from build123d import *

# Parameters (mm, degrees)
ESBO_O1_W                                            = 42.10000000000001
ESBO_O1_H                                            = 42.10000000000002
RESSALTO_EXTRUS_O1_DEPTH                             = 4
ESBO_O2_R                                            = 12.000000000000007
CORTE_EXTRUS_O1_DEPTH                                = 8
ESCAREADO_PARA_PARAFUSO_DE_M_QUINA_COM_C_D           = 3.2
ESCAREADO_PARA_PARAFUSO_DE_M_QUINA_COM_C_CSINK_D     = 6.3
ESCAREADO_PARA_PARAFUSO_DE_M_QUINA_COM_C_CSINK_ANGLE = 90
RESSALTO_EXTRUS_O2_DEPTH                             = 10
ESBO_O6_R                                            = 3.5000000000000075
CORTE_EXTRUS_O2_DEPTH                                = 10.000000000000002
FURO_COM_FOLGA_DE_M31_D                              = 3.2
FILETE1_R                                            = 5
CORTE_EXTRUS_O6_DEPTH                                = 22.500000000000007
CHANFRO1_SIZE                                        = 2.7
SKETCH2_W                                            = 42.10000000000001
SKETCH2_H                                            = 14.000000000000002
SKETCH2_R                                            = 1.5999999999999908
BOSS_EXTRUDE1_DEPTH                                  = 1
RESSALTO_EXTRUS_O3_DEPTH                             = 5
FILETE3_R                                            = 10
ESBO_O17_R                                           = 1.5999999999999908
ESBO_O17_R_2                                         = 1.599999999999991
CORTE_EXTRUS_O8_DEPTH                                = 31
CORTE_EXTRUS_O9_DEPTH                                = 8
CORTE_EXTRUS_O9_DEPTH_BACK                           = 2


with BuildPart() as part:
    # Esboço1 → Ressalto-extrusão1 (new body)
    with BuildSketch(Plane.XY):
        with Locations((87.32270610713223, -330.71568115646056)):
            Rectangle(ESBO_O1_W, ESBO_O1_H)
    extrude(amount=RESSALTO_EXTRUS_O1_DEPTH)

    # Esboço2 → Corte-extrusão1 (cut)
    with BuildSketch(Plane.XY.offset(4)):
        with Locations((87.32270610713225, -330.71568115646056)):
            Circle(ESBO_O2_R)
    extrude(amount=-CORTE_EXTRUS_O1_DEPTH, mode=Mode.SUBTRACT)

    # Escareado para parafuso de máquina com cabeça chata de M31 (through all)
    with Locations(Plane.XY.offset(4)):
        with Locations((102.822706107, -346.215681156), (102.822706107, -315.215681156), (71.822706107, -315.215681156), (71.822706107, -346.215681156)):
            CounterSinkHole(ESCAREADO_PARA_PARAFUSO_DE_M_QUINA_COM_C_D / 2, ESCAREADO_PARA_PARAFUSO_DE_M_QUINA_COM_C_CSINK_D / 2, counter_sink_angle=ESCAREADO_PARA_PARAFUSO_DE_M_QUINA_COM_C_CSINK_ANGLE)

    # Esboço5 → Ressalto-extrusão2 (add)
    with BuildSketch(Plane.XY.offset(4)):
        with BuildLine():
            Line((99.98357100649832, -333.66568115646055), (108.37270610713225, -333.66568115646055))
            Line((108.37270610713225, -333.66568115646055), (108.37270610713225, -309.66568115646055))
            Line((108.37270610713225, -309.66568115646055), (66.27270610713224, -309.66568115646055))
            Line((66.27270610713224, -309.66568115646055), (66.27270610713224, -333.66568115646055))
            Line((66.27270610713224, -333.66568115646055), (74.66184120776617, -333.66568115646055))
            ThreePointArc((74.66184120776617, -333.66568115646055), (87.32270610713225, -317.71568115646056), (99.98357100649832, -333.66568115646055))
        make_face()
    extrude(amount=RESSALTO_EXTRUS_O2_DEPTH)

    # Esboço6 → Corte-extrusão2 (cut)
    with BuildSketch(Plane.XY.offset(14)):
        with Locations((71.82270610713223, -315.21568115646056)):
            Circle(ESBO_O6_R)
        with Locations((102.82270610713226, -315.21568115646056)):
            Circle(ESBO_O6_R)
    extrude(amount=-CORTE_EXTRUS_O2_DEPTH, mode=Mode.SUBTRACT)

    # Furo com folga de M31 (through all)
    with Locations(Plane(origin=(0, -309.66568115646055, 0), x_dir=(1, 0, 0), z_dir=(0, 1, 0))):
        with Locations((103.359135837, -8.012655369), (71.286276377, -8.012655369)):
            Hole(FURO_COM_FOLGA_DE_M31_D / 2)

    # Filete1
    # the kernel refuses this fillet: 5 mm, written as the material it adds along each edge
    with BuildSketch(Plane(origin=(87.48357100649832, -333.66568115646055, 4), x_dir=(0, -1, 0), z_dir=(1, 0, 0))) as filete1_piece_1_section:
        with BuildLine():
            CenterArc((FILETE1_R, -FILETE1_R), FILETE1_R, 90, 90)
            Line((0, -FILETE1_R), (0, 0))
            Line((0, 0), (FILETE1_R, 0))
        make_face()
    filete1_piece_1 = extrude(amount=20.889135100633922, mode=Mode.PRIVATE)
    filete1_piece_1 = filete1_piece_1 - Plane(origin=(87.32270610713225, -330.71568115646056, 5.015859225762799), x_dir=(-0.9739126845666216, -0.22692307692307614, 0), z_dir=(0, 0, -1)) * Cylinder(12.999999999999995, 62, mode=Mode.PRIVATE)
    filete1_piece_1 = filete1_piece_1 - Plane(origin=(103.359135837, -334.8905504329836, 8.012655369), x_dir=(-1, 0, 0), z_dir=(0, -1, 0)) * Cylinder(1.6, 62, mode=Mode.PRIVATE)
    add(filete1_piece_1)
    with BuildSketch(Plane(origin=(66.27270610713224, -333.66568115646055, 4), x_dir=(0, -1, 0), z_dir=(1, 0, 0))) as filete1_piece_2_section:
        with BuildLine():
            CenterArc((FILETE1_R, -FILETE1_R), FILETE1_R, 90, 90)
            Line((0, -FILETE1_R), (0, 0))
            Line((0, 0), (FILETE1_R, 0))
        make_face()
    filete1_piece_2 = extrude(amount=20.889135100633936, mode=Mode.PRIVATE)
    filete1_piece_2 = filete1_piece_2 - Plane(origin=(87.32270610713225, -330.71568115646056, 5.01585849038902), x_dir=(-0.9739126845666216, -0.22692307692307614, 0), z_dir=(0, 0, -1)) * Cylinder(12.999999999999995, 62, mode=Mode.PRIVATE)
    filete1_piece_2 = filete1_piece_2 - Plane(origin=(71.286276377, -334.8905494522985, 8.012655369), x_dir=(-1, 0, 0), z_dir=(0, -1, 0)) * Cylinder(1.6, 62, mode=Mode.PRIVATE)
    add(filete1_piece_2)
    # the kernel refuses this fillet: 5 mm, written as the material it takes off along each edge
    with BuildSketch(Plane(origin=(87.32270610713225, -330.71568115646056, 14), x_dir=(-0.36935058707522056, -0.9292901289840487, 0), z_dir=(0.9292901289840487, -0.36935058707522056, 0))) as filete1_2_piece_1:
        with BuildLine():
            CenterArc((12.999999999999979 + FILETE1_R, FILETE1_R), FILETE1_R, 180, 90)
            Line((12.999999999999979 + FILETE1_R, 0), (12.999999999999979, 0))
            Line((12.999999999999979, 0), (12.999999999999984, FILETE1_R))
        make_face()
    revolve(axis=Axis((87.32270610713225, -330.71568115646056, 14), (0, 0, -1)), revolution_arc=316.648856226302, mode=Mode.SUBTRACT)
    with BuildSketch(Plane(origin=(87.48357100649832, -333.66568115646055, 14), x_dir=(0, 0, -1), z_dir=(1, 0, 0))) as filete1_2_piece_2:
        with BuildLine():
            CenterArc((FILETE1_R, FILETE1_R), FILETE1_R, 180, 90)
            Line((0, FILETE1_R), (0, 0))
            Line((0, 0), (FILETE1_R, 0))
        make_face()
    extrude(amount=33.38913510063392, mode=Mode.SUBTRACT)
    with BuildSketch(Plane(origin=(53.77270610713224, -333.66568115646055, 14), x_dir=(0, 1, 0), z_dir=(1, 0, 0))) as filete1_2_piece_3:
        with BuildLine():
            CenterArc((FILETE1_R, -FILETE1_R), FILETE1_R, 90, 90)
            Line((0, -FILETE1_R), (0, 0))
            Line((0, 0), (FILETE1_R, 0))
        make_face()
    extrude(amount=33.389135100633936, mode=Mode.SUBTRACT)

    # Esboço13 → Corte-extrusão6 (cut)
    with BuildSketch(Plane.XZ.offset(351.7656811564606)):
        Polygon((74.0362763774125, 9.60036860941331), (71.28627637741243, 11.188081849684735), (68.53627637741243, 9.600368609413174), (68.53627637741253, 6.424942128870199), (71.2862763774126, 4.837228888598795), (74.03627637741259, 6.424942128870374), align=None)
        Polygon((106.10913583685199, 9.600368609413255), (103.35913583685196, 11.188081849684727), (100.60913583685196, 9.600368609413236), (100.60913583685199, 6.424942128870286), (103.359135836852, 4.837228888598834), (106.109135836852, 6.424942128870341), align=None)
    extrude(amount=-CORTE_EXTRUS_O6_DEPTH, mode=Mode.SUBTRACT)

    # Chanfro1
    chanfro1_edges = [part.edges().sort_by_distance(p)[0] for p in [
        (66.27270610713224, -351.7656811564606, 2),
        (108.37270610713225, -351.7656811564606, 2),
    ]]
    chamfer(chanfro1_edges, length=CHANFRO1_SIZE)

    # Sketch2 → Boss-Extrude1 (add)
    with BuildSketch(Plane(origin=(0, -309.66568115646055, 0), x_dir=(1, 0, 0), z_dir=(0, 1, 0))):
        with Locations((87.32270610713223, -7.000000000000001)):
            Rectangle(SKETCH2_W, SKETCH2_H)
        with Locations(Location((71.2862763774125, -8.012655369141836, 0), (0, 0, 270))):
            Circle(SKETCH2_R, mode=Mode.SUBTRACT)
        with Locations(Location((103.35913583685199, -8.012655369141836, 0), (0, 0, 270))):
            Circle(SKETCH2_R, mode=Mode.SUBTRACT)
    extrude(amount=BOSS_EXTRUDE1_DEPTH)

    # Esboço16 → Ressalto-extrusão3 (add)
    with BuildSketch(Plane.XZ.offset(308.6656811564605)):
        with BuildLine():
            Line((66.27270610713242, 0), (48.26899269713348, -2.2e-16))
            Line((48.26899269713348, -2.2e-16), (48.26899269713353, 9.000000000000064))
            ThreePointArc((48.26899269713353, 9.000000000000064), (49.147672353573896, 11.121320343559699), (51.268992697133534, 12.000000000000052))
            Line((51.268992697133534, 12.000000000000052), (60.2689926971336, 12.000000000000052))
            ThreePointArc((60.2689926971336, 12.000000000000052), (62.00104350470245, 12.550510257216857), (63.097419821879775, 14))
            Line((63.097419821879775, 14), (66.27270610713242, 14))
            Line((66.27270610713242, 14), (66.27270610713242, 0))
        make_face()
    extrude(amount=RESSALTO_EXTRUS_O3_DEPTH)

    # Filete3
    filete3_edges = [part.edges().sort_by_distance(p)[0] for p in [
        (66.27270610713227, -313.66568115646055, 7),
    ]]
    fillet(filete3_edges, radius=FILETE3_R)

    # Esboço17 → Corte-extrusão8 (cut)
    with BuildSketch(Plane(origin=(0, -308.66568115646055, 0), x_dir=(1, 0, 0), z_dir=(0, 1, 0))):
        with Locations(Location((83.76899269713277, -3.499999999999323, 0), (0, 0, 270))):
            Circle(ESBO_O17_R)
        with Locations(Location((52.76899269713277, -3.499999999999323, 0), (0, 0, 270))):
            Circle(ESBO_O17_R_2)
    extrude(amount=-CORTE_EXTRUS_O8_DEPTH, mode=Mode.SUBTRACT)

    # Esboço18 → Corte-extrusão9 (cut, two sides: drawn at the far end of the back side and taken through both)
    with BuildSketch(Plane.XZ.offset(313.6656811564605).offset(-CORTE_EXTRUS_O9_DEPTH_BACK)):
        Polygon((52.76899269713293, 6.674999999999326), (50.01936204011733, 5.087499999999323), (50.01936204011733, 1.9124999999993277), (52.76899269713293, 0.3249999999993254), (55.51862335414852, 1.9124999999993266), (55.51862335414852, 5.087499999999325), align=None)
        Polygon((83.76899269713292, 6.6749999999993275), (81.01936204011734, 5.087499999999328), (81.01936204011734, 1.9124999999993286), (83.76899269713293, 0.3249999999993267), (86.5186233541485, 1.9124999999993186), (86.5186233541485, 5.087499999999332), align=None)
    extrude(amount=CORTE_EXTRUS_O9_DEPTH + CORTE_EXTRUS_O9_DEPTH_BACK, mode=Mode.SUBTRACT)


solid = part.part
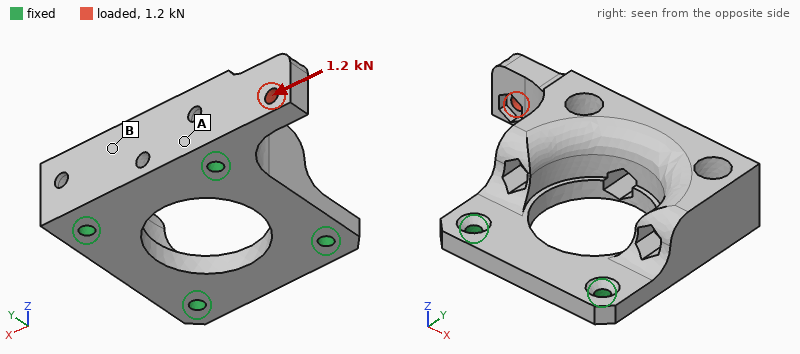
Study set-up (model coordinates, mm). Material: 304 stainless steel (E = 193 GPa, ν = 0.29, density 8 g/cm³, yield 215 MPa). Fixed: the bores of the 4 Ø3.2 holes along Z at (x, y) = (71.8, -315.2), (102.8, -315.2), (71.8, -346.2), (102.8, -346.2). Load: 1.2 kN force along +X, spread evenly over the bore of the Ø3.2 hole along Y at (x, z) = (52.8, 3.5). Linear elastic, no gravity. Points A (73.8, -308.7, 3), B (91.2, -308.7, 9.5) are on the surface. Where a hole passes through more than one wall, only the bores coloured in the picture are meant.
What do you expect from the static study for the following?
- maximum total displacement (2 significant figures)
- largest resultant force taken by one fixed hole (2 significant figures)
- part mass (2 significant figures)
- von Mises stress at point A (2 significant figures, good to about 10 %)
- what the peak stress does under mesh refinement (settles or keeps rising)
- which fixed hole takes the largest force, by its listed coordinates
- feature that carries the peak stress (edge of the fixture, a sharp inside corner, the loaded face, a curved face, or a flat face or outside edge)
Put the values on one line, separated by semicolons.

14 µm; 980 N; 96 g; 20 MPa; keeps rising; (71.8, -315.2); edge of the fixture
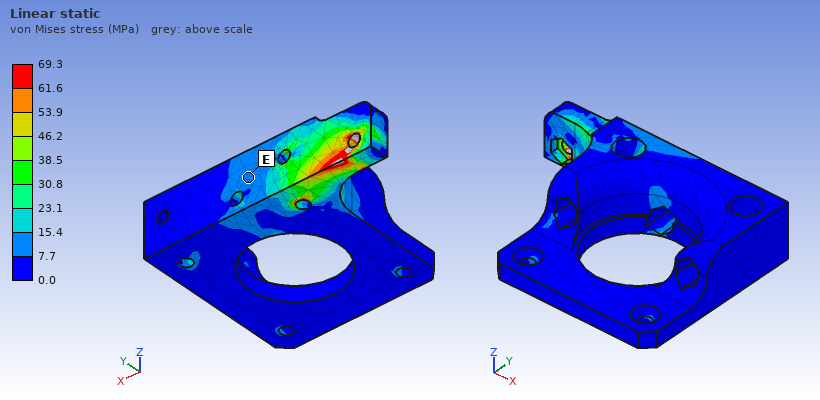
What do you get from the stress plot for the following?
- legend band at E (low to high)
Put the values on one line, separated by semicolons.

7.7 to 15.4 MPa
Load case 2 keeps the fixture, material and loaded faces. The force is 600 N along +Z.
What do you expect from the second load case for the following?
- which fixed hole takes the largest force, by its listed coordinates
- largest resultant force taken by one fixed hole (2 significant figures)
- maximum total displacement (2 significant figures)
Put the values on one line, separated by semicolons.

(71.8, -315.2); 1.1 kN; 18 µm
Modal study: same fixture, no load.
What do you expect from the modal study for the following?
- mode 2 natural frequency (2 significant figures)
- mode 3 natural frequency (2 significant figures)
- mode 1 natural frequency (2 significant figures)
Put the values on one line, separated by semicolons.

13 kHz; 14 kHz; 12 kHz
